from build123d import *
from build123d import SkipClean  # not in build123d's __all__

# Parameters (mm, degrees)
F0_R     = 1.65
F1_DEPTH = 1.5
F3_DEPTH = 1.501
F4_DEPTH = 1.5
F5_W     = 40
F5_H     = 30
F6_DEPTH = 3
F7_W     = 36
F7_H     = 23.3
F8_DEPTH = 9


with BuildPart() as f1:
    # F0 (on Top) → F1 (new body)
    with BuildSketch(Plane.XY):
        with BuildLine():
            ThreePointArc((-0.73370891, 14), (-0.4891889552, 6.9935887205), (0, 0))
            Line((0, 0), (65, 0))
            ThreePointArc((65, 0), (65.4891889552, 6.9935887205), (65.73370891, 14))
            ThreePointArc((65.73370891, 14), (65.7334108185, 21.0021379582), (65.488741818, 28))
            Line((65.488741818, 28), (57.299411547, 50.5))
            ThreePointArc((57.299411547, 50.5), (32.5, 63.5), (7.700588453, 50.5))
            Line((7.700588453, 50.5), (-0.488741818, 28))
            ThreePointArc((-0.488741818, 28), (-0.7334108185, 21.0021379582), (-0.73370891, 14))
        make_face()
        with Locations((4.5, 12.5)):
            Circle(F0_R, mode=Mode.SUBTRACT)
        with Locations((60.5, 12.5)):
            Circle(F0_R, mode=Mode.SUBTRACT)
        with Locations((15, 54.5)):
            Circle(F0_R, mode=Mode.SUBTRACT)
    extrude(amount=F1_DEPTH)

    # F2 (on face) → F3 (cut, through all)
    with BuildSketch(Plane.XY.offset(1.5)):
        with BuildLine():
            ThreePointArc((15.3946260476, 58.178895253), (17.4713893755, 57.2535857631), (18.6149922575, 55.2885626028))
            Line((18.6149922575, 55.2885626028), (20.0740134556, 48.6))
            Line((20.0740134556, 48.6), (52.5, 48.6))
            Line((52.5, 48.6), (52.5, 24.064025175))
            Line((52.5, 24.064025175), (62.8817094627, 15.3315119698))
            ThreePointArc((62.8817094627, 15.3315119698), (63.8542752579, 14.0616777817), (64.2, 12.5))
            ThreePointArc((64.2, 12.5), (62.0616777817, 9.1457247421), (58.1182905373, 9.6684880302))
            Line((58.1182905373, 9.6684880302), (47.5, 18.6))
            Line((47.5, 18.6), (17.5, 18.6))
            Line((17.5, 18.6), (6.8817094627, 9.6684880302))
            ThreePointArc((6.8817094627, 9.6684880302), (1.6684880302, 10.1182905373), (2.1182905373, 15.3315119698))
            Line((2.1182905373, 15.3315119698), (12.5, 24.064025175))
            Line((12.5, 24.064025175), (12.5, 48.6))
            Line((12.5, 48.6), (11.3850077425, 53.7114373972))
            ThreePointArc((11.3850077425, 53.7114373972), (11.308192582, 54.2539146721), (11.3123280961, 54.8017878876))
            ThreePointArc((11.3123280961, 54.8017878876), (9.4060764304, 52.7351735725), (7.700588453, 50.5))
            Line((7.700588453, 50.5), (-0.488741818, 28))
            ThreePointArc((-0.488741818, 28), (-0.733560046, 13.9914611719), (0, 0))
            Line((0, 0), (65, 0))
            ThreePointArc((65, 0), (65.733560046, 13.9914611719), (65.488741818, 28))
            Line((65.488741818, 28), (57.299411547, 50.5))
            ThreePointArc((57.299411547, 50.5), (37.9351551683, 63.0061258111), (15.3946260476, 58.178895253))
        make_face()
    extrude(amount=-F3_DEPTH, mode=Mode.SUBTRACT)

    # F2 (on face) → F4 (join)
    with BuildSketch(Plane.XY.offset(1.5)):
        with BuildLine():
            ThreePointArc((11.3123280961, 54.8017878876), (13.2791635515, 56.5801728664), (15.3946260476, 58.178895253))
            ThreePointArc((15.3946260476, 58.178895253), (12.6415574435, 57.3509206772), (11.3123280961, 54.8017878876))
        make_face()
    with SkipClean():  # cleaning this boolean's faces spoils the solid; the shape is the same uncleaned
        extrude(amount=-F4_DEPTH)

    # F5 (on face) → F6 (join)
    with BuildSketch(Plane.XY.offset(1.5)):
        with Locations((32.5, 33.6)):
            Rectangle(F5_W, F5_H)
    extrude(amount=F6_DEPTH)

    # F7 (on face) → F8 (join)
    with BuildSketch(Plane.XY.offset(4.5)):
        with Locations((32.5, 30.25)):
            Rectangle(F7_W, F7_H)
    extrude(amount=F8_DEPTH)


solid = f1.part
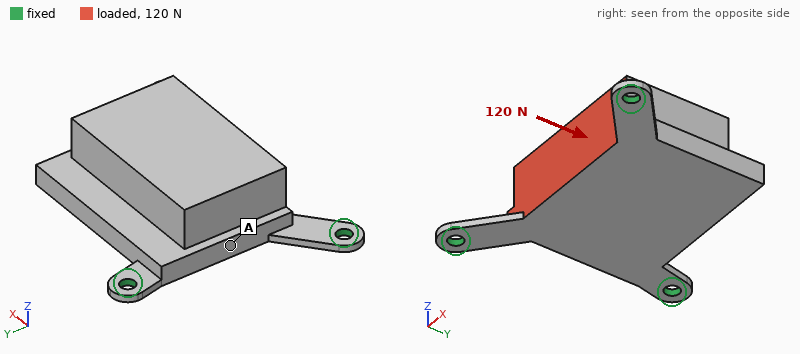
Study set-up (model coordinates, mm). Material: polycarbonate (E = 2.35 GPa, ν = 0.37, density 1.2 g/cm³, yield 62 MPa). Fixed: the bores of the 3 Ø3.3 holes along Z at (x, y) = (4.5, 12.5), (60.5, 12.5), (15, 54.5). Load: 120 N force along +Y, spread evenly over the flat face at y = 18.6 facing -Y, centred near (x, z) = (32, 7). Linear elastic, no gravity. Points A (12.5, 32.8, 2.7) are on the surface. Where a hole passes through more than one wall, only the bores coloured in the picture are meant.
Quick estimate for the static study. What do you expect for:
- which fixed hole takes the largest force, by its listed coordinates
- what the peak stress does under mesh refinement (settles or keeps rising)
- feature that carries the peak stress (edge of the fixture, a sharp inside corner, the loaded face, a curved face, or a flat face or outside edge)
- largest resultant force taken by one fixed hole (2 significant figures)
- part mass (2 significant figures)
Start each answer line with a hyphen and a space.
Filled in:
- (15, 54.5)
- keeps rising
- edge of the fixture
- 65 N
- 16 g
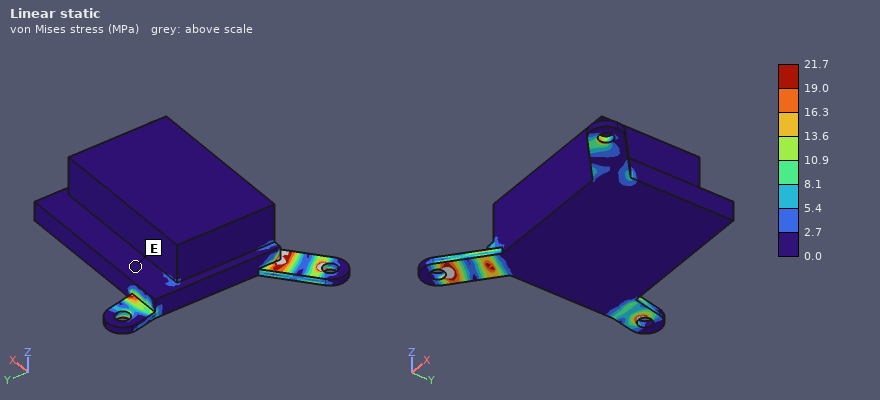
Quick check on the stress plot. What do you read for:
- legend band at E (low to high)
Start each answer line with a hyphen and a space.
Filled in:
- 0.0 to 2.7 MPa
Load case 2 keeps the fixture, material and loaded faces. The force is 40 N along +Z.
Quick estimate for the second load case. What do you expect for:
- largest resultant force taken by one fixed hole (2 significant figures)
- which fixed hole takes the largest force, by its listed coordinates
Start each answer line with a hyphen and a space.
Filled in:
- 22 N
- (60.5, 12.5)
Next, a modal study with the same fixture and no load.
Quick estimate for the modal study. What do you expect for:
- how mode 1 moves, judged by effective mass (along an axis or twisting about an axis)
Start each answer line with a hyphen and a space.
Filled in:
- along Z
